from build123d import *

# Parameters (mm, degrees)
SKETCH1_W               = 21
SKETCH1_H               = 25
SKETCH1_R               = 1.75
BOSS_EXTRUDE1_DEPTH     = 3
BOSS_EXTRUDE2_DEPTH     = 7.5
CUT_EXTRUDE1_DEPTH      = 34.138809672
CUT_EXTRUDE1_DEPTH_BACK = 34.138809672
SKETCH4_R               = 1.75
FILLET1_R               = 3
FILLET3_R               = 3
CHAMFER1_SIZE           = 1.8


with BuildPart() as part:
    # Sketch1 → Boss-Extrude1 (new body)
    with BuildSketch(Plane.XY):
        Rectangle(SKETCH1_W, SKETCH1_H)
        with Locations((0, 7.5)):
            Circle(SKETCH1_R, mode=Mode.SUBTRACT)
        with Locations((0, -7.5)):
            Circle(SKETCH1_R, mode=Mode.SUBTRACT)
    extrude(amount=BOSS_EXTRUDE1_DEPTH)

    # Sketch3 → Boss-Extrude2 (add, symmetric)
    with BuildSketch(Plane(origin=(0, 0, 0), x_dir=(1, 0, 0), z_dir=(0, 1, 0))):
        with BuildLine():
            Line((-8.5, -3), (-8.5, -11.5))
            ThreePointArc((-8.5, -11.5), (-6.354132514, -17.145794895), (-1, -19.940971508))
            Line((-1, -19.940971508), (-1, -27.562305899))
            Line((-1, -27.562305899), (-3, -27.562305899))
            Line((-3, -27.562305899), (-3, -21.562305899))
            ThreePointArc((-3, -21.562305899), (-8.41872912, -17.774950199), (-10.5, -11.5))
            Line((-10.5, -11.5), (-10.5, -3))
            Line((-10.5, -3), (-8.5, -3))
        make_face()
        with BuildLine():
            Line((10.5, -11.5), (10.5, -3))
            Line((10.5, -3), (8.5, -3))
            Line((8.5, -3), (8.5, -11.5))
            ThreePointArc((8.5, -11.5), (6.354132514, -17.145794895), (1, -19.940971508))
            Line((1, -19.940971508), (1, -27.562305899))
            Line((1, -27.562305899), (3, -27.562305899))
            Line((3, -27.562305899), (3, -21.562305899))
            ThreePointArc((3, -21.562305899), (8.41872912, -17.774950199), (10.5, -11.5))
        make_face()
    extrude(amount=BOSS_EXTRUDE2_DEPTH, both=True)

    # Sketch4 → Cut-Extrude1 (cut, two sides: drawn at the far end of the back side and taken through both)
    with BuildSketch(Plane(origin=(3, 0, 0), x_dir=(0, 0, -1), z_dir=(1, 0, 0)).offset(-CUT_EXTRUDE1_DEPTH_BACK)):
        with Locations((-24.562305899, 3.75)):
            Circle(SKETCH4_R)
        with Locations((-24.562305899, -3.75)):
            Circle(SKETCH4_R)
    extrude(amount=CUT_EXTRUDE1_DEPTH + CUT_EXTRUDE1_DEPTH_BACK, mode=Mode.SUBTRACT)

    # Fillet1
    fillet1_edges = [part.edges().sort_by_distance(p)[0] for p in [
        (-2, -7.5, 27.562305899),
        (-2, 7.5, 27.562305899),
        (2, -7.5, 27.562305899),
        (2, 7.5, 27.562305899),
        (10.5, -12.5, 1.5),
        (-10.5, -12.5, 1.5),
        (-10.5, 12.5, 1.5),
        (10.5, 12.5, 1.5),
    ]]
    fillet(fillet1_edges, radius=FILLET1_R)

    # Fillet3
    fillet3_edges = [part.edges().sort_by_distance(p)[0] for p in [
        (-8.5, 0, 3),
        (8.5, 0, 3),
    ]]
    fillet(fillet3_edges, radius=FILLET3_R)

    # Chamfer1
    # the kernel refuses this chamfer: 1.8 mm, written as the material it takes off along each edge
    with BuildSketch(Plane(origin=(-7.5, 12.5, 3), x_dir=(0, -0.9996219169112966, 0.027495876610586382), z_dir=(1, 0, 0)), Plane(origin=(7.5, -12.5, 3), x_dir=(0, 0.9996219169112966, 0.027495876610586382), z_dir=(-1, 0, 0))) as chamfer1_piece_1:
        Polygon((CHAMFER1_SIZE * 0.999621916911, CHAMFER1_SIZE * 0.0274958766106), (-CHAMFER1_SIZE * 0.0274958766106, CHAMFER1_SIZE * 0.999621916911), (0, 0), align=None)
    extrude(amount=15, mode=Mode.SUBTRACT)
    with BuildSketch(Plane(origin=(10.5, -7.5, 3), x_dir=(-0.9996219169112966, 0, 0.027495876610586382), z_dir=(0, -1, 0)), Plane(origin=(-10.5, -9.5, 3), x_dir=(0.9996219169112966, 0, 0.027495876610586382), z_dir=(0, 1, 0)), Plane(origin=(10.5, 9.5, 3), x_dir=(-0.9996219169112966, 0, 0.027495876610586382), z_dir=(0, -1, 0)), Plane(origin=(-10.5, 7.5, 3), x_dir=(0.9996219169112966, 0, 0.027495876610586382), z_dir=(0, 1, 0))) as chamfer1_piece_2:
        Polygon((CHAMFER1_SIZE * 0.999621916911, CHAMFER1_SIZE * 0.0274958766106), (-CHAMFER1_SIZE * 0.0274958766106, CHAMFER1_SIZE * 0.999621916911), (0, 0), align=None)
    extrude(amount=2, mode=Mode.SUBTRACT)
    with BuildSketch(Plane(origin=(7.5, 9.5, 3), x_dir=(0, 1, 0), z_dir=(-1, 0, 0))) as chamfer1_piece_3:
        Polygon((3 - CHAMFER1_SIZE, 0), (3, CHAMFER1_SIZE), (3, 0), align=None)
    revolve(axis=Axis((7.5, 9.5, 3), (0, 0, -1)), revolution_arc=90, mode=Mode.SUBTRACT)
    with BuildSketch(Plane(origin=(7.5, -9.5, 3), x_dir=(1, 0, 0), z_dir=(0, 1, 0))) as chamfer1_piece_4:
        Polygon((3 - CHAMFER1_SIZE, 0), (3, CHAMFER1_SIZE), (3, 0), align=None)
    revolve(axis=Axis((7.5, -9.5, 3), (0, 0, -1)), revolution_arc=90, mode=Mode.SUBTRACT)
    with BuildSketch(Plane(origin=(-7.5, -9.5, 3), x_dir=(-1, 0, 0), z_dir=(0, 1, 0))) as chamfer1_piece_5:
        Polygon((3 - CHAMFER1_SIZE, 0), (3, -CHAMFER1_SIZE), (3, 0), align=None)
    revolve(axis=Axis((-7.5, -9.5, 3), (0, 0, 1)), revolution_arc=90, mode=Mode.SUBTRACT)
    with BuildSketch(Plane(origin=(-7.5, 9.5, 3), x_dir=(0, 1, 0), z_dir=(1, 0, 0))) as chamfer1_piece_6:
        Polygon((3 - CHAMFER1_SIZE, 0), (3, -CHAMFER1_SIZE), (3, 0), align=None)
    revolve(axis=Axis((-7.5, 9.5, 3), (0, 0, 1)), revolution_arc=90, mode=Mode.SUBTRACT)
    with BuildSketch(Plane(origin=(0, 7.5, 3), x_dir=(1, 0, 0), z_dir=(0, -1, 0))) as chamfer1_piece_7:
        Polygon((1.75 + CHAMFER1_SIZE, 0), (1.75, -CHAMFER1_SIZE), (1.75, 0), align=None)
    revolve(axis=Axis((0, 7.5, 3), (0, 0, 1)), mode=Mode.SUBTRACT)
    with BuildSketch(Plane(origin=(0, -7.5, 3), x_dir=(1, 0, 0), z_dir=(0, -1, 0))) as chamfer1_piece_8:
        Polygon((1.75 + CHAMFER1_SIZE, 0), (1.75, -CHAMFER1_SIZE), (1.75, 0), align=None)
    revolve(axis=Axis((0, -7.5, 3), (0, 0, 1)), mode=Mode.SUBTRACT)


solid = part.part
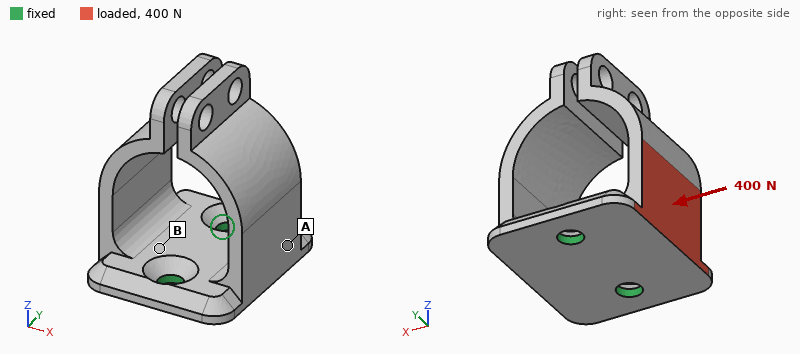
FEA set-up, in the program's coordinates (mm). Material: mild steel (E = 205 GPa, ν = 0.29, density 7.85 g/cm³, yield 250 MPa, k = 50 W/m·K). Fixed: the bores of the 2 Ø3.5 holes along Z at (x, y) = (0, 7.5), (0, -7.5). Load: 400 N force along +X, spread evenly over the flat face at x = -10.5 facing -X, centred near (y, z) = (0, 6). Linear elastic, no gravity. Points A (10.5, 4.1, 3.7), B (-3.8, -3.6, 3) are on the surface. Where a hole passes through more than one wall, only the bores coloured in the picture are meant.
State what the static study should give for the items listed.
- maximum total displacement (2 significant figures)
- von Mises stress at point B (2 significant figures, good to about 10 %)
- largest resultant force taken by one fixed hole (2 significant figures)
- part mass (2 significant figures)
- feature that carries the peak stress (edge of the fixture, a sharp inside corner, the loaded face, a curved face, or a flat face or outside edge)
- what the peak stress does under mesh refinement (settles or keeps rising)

82 µm
63 MPa
200 N
24 g
edge of the fixture
keeps rising
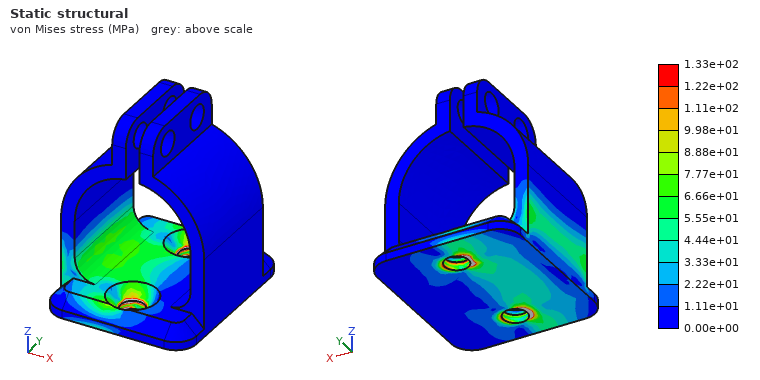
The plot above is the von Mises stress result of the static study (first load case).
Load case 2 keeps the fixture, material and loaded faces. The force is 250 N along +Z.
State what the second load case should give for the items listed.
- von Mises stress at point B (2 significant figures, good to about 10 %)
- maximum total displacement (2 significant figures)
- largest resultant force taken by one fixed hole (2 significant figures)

60 MPa
62 µm
150 N
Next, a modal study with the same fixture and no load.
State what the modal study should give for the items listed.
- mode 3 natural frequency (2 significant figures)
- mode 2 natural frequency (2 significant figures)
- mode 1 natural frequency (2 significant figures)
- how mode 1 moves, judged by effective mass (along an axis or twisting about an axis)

4700 Hz
2300 Hz
2200 Hz
along X
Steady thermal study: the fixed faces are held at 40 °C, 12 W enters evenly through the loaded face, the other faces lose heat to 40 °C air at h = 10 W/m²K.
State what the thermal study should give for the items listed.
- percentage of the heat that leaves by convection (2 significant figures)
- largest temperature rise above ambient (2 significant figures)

5.4 %
59 K
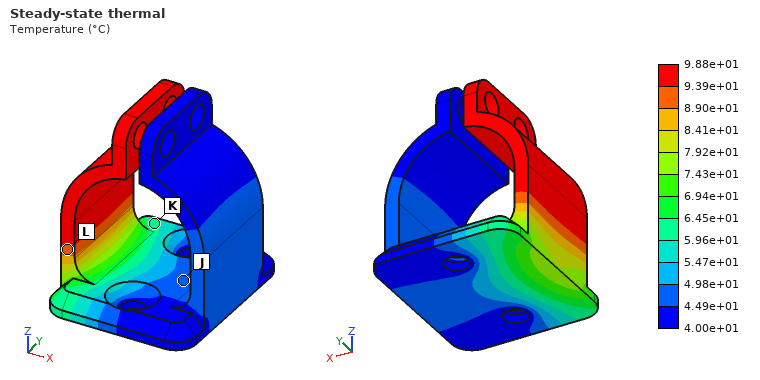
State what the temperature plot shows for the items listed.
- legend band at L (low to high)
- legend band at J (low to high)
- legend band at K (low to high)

8.90e+01 to 9.39e+01 °C
4.49e+01 to 4.98e+01 °C
5.96e+01 to 6.45e+01 °C
